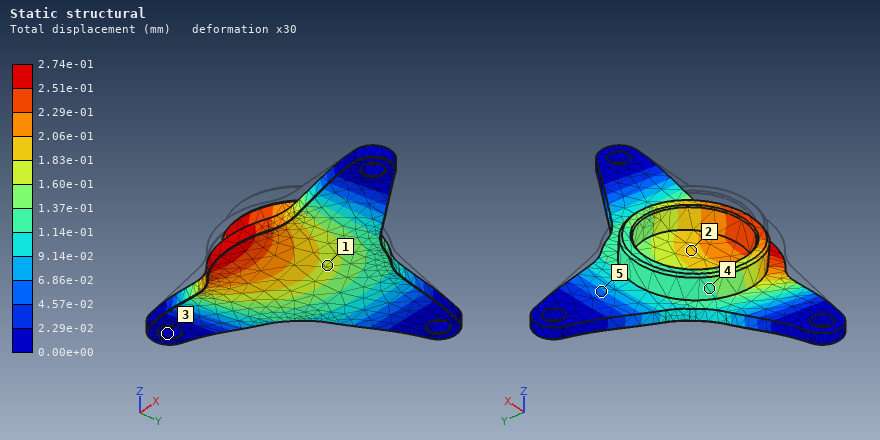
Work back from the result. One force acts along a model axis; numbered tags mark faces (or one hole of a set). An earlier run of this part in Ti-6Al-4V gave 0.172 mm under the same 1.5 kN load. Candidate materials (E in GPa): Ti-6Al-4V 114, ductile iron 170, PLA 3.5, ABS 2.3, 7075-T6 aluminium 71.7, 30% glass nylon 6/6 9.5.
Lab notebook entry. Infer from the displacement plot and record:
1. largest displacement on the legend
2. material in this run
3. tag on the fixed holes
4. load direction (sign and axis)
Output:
2.74e-01 mm
7075-T6 aluminium
3
-Z
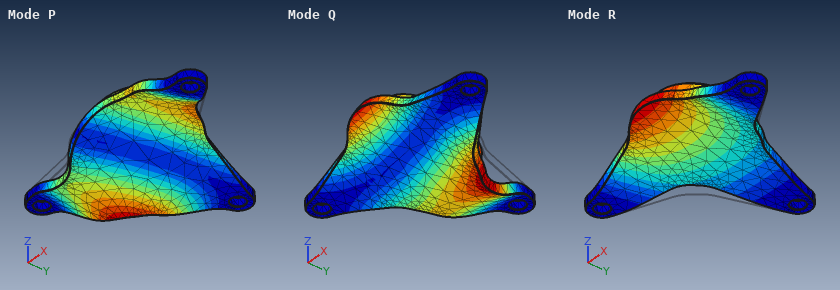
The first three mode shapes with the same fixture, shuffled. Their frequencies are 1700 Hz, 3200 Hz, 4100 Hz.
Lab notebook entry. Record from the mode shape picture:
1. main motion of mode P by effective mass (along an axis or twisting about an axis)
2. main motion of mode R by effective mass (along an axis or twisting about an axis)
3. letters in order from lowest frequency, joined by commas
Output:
twisting about Y
along Z
R, Q, P
